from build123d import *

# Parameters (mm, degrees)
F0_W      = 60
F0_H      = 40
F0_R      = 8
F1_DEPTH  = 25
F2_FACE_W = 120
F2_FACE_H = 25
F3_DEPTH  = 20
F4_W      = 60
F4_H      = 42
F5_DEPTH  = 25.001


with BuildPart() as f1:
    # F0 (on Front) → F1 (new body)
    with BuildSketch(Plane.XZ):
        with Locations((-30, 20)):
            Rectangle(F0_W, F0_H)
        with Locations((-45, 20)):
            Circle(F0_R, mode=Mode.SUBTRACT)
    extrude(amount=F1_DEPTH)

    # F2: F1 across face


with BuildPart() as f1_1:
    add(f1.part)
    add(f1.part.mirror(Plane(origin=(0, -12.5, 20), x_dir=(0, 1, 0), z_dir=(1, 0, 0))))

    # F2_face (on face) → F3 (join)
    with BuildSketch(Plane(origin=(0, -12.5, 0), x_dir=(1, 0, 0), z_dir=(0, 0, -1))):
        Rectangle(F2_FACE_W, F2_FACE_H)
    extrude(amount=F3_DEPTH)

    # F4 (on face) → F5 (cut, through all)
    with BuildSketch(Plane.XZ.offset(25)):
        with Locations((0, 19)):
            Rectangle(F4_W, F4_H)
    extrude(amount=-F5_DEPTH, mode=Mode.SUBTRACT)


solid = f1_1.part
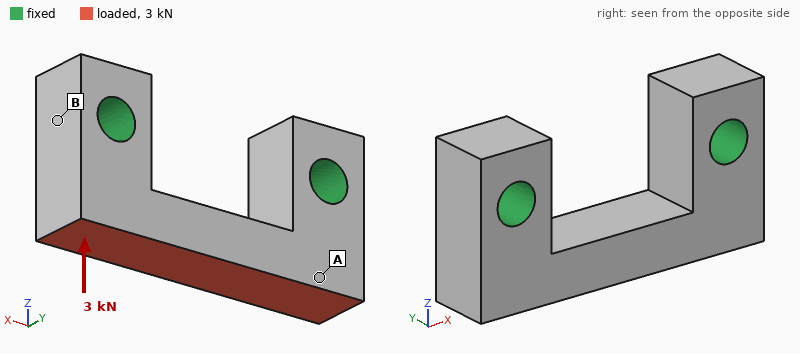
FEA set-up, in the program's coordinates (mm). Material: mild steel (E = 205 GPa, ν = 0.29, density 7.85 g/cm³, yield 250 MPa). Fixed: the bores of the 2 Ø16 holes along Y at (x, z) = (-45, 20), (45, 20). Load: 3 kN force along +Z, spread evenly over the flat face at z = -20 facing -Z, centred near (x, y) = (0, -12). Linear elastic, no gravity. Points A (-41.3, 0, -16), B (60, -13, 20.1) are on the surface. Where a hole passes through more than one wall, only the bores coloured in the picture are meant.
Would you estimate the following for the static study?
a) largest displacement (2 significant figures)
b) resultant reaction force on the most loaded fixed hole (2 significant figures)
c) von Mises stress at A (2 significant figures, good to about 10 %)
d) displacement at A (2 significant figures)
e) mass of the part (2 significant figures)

1.7 µm
1.6 kN
1.7 MPa
0.33 µm
840 g
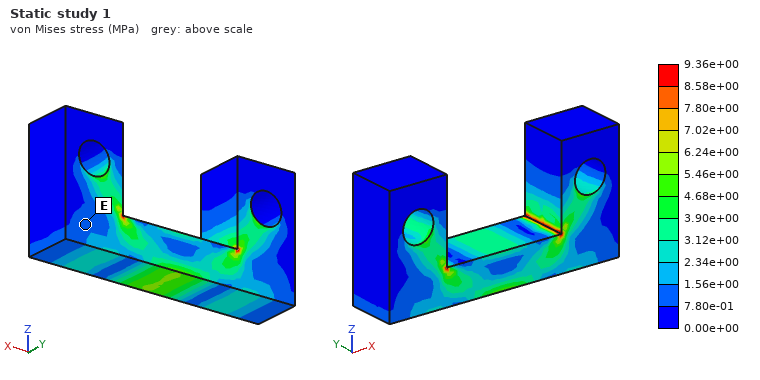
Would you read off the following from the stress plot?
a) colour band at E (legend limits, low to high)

7.80e-01 to 1.56e+00 MPa
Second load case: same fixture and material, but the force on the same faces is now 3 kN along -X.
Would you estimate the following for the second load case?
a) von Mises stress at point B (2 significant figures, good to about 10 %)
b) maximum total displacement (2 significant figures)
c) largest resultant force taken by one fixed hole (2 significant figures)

3.7 MPa
2.3 µm
1.6 kN
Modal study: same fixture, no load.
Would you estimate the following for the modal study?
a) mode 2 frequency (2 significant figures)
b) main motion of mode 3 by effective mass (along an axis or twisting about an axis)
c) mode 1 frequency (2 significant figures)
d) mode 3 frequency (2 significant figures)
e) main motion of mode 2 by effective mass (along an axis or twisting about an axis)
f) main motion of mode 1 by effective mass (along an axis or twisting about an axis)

10 kHz
along Z
7700 Hz
11 kHz
along X
along Y
